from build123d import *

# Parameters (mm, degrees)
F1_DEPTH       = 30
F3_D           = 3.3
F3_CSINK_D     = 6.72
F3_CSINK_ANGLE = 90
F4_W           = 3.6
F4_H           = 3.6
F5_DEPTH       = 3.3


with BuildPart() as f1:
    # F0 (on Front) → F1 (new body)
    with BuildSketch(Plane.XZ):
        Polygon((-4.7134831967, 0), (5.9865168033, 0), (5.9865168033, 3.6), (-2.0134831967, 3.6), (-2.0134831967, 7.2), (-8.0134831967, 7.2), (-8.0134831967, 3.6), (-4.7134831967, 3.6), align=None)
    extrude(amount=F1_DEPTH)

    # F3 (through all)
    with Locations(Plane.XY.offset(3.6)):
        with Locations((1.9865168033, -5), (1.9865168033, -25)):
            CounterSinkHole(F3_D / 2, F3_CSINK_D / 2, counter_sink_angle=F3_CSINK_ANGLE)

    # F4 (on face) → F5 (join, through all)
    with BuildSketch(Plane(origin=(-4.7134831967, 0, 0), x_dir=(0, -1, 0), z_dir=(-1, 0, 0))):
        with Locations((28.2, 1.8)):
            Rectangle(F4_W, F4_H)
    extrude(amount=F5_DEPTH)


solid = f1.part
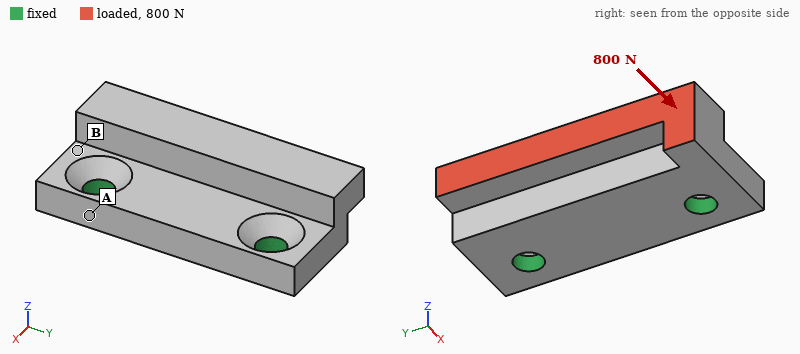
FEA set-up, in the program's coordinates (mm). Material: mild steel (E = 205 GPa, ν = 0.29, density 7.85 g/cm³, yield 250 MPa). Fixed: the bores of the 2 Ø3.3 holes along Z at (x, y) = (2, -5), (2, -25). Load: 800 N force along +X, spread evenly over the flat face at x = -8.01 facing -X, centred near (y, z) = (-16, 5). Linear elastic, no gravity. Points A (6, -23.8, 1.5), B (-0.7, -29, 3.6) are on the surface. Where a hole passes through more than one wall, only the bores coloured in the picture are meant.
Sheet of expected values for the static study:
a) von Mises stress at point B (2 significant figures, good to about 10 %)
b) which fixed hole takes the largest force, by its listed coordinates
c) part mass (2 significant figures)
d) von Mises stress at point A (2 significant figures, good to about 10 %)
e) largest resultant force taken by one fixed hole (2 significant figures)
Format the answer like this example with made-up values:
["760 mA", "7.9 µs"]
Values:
["70 MPa", "(2, -25)", "14 g", "34 MPa", "450 N"]
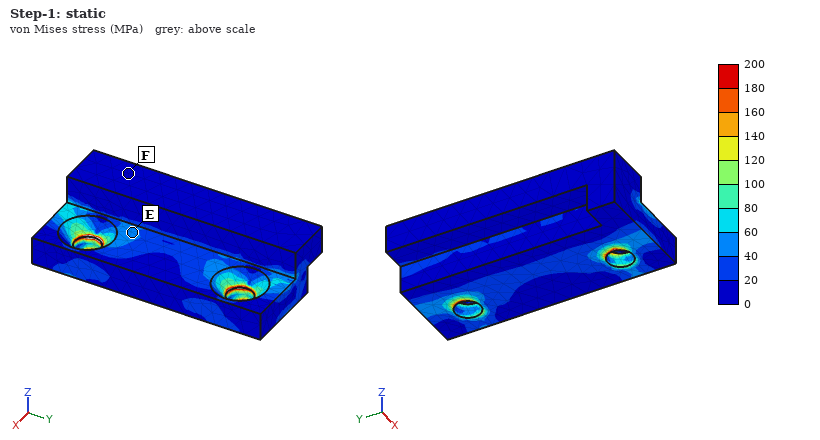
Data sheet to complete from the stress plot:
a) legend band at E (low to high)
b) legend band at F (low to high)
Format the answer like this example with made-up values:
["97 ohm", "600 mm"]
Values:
["40 to 60 MPa", "0 to 20 MPa"]
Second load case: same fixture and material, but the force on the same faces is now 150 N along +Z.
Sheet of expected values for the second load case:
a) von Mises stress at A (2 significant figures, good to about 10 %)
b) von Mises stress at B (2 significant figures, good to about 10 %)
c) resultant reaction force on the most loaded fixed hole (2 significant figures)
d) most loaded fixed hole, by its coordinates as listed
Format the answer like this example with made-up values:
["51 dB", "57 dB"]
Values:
["13 MPa", "28 MPa", "86 N", "(2, -25)"]
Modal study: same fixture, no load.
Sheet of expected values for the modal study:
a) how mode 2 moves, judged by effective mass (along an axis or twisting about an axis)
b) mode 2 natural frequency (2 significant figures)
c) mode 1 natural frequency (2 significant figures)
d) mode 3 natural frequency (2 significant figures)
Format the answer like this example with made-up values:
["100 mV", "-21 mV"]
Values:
["twisting about X", "22 kHz", "13 kHz", "35 kHz"]
